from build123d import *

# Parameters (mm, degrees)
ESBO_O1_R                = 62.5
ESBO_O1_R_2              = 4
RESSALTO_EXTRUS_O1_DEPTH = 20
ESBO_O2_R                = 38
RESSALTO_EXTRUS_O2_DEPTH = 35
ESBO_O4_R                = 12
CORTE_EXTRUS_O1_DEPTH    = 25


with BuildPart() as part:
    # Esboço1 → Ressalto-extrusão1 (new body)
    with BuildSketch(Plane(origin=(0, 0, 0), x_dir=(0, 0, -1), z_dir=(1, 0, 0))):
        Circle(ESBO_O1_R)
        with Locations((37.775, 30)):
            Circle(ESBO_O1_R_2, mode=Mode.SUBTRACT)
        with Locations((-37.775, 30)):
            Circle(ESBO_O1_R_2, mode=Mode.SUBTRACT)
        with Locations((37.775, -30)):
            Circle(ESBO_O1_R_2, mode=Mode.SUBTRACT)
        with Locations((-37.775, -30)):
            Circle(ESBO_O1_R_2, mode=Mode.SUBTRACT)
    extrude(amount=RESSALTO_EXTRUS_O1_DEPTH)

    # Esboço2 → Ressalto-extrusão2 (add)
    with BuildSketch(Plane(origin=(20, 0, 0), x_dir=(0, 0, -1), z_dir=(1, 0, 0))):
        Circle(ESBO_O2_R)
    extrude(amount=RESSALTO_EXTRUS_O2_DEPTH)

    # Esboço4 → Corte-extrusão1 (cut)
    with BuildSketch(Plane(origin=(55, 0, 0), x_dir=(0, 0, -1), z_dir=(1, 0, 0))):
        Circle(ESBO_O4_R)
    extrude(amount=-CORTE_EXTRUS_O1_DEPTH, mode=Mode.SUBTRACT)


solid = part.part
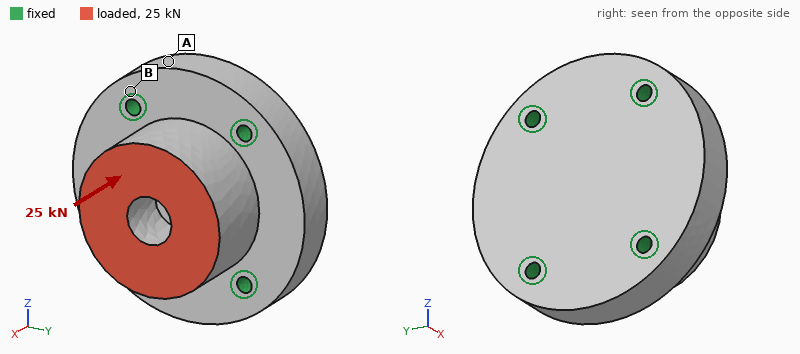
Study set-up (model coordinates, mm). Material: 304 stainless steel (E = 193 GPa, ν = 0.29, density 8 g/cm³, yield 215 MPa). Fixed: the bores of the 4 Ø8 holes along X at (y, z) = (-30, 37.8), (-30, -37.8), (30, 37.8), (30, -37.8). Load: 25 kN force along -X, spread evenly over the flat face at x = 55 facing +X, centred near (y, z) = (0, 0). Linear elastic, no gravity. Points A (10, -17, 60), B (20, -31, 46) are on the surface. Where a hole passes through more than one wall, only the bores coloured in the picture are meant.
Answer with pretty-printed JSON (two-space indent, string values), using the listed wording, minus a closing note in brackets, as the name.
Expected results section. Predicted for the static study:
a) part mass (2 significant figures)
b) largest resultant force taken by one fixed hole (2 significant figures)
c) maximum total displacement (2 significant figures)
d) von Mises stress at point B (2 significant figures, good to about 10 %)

{
  "part mass": "3.1 kg",
  "largest resultant force taken by one fixed hole": "6.5 kN",
  "maximum total displacement": "4.5 µm",
  "von Mises stress at point B": "8.8 MPa"
}
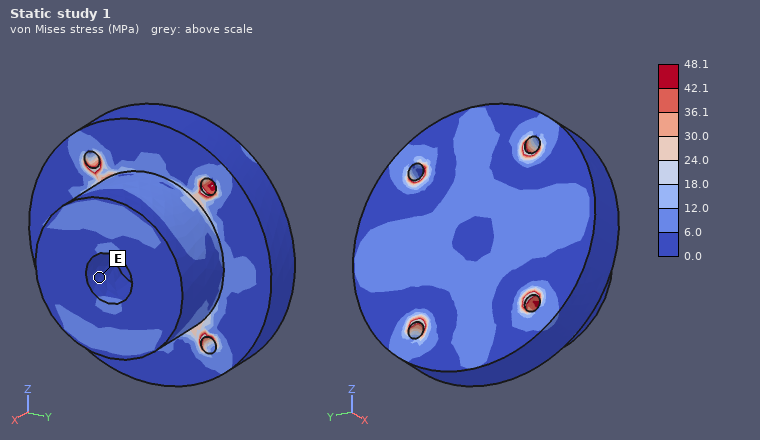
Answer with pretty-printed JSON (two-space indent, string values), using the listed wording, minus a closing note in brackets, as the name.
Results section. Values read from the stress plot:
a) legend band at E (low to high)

{
  "legend band at E": "0.0 to 6.0 MPa"
}
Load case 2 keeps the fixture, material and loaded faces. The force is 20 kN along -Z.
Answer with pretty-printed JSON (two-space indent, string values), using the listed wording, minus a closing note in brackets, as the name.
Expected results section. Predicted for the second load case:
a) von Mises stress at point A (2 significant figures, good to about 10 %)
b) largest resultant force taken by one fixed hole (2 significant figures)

{
  "von Mises stress at point A": "5.7 MPa",
  "largest resultant force taken by one fixed hole": "8.0 kN"
}
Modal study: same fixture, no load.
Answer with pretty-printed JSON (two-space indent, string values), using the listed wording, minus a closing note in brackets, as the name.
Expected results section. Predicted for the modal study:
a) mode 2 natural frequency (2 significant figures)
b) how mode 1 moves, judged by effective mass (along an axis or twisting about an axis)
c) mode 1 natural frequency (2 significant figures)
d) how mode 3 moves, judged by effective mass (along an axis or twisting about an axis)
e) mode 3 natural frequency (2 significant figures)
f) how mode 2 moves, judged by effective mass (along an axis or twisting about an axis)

{
  "mode 2 natural frequency": "8900 Hz",
  "how mode 1 moves, judged by effective mass": "along Y",
  "mode 1 natural frequency": "7600 Hz",
  "how mode 3 moves, judged by effective mass": "along Z",
  "mode 3 natural frequency": "9600 Hz",
  "how mode 2 moves, judged by effective mass": "along X"
}
